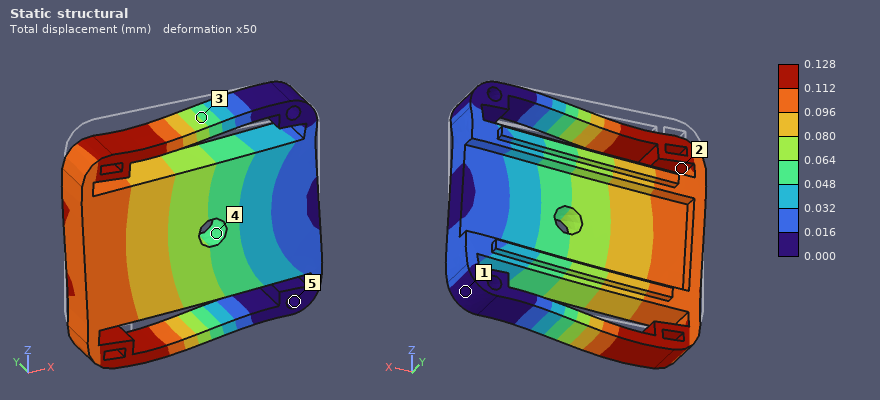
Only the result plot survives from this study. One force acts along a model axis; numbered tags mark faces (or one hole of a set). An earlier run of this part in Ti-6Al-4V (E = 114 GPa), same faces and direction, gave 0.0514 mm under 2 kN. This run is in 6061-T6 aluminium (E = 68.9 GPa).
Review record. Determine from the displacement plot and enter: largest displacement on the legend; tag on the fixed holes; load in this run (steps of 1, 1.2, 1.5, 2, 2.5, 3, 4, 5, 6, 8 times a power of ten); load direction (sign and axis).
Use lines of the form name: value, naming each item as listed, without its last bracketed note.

largest displacement on the legend: 0.128 mm
tag on the fixed holes: 5
load in this run: 3 kN
load direction: -Z
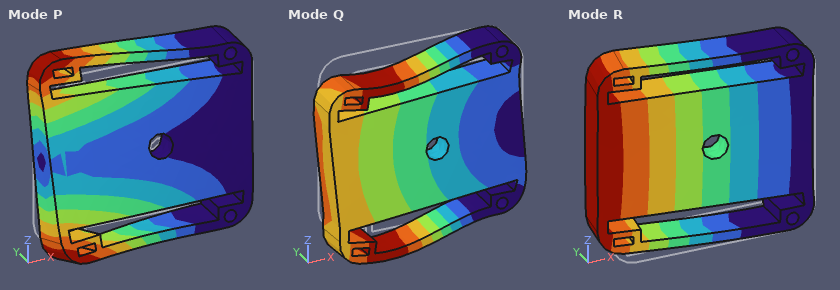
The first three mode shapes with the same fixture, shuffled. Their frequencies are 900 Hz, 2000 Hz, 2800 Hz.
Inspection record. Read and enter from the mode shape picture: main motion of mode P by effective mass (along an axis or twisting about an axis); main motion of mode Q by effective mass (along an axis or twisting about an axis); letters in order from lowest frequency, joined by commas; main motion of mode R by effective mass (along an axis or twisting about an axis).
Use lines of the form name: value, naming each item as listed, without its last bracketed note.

main motion of mode P by effective mass: twisting about X
main motion of mode Q by effective mass: along Z
letters in order from lowest frequency, joined by commas: R, Q, P
main motion of mode R by effective mass: along Y
